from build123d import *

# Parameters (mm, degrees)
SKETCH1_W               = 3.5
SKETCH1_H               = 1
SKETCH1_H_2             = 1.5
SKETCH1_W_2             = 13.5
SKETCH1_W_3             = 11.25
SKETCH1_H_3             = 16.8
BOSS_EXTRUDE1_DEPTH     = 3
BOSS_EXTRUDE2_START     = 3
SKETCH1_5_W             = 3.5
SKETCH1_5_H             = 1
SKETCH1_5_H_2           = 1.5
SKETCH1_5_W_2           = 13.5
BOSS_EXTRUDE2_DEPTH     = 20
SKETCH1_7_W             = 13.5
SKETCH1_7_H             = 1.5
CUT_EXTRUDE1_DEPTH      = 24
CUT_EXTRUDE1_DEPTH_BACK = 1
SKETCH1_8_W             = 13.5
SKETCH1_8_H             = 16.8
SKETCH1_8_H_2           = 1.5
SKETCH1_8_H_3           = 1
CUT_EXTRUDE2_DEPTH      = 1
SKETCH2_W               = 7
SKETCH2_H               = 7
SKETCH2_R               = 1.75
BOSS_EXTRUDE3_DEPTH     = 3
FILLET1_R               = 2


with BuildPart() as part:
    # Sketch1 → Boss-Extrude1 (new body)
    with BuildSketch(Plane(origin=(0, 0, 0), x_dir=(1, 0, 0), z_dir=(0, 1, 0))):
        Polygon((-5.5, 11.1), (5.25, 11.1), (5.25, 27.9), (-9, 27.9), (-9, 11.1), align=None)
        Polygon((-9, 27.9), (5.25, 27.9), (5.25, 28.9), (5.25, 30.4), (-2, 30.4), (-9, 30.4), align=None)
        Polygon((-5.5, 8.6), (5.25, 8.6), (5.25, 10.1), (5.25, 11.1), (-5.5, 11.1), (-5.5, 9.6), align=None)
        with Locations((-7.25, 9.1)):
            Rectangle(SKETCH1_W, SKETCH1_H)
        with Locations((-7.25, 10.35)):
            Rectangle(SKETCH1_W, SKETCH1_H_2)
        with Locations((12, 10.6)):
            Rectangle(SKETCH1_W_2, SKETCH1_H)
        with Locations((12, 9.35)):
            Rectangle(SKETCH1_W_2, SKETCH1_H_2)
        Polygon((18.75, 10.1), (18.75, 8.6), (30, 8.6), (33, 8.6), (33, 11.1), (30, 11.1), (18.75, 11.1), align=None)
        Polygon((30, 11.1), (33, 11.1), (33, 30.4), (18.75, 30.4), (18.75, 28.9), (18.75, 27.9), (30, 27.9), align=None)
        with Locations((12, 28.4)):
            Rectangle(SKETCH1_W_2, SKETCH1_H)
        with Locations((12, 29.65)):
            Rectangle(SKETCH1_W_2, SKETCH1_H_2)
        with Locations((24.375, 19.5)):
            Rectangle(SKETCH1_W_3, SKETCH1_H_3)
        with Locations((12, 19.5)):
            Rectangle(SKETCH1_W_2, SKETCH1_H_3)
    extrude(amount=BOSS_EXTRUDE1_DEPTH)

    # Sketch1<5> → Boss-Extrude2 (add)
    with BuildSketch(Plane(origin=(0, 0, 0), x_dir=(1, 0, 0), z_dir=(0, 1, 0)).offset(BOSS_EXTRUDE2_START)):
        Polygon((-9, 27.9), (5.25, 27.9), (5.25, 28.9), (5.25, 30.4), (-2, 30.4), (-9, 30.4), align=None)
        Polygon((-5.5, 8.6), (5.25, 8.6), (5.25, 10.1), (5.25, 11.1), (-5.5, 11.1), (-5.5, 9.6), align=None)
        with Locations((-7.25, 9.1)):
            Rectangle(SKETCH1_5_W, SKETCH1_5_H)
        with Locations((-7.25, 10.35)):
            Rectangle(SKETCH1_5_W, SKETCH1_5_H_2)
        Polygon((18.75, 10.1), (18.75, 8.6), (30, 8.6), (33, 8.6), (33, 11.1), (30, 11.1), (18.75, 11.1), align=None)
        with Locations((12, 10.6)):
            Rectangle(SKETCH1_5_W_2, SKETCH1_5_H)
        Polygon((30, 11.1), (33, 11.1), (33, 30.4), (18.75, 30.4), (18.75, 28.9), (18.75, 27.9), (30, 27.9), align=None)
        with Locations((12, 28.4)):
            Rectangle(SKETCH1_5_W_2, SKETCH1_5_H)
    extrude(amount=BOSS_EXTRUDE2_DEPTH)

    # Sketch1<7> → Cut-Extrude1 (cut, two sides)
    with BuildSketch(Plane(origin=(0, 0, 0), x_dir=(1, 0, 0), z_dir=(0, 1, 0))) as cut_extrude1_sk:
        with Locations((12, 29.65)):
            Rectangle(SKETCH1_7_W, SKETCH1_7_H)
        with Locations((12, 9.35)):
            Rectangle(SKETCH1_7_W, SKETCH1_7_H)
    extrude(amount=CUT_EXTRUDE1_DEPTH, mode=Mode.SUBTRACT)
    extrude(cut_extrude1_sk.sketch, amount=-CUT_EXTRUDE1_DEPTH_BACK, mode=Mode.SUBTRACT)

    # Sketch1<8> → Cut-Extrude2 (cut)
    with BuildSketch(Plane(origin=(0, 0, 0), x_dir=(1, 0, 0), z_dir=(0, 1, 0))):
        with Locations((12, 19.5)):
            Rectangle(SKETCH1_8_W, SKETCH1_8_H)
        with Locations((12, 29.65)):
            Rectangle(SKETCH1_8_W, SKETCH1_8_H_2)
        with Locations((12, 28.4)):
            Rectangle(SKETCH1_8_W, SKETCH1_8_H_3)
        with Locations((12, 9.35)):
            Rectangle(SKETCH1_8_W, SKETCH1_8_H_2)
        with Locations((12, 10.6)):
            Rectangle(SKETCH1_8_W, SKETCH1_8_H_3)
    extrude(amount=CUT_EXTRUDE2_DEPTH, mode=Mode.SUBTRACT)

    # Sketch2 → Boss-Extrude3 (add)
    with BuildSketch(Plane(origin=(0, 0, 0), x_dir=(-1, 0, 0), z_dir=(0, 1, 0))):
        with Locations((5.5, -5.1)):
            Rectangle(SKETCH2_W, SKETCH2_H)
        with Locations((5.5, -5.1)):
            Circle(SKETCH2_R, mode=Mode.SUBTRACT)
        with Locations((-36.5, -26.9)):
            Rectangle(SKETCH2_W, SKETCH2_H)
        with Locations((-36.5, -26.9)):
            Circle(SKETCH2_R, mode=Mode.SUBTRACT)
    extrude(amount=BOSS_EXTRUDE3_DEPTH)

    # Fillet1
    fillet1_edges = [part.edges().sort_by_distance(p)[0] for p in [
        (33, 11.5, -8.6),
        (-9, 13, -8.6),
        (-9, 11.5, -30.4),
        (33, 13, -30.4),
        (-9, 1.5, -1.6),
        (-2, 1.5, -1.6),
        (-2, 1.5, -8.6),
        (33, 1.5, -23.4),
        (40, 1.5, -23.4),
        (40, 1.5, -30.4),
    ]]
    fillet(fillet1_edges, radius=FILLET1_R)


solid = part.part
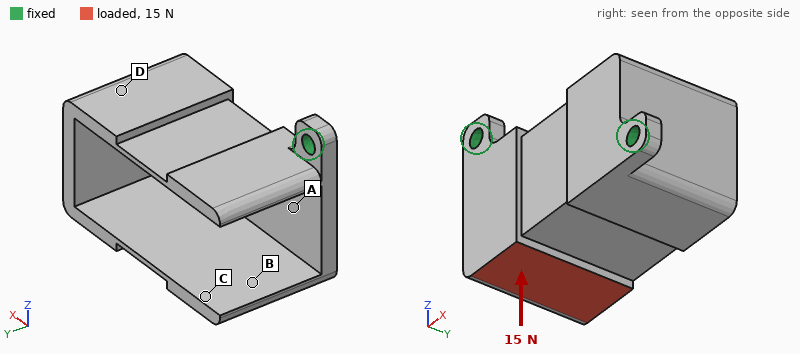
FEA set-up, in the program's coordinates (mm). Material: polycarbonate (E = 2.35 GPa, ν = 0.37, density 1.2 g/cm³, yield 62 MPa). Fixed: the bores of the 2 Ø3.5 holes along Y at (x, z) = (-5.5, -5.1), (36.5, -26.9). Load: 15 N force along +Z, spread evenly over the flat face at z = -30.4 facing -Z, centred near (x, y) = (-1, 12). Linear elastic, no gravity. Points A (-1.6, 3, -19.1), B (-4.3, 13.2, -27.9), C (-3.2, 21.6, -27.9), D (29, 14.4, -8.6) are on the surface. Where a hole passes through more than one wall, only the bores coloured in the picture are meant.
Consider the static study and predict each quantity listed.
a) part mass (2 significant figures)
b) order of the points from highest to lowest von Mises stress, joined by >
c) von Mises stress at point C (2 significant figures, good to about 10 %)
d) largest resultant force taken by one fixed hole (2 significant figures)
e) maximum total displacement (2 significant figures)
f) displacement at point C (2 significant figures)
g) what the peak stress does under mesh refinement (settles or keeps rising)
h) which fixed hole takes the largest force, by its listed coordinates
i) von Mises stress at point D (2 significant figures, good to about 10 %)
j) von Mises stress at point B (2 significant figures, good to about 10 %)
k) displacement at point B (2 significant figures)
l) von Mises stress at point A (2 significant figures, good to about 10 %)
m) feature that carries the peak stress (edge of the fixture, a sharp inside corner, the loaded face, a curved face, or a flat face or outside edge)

8.3 g
A > B > C > D
1.1 MPa
13 N
0.72 mm
0.62 mm
keeps rising
(-5.5, -5.1)
0.58 MPa
1.9 MPa
0.36 mm
3.0 MPa
edge of the fixture
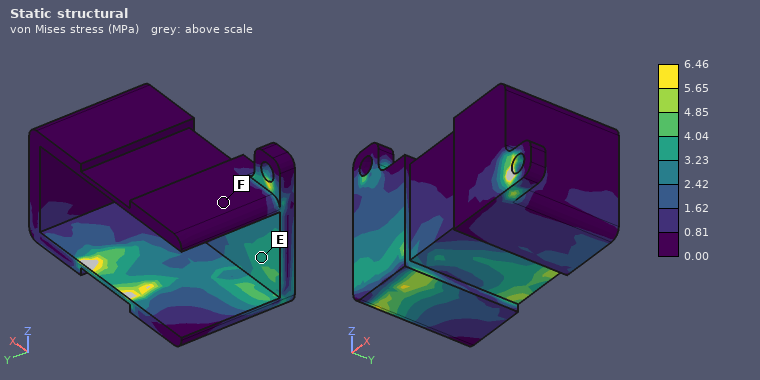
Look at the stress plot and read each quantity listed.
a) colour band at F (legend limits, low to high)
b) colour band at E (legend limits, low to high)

0.00 to 0.81 MPa
3.23 to 4.04 MPa
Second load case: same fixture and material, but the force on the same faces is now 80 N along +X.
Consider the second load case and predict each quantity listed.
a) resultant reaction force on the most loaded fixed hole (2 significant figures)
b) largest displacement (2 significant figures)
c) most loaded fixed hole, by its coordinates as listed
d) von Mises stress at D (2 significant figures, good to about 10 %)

67 N
0.71 mm
(36.5, -26.9)
2.2 MPa
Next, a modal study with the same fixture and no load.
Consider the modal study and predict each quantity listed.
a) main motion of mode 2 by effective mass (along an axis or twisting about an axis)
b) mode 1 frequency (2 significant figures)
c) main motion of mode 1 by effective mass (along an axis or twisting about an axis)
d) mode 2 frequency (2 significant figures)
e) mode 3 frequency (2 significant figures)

along Y
580 Hz
along Z
980 Hz
1100 Hz
